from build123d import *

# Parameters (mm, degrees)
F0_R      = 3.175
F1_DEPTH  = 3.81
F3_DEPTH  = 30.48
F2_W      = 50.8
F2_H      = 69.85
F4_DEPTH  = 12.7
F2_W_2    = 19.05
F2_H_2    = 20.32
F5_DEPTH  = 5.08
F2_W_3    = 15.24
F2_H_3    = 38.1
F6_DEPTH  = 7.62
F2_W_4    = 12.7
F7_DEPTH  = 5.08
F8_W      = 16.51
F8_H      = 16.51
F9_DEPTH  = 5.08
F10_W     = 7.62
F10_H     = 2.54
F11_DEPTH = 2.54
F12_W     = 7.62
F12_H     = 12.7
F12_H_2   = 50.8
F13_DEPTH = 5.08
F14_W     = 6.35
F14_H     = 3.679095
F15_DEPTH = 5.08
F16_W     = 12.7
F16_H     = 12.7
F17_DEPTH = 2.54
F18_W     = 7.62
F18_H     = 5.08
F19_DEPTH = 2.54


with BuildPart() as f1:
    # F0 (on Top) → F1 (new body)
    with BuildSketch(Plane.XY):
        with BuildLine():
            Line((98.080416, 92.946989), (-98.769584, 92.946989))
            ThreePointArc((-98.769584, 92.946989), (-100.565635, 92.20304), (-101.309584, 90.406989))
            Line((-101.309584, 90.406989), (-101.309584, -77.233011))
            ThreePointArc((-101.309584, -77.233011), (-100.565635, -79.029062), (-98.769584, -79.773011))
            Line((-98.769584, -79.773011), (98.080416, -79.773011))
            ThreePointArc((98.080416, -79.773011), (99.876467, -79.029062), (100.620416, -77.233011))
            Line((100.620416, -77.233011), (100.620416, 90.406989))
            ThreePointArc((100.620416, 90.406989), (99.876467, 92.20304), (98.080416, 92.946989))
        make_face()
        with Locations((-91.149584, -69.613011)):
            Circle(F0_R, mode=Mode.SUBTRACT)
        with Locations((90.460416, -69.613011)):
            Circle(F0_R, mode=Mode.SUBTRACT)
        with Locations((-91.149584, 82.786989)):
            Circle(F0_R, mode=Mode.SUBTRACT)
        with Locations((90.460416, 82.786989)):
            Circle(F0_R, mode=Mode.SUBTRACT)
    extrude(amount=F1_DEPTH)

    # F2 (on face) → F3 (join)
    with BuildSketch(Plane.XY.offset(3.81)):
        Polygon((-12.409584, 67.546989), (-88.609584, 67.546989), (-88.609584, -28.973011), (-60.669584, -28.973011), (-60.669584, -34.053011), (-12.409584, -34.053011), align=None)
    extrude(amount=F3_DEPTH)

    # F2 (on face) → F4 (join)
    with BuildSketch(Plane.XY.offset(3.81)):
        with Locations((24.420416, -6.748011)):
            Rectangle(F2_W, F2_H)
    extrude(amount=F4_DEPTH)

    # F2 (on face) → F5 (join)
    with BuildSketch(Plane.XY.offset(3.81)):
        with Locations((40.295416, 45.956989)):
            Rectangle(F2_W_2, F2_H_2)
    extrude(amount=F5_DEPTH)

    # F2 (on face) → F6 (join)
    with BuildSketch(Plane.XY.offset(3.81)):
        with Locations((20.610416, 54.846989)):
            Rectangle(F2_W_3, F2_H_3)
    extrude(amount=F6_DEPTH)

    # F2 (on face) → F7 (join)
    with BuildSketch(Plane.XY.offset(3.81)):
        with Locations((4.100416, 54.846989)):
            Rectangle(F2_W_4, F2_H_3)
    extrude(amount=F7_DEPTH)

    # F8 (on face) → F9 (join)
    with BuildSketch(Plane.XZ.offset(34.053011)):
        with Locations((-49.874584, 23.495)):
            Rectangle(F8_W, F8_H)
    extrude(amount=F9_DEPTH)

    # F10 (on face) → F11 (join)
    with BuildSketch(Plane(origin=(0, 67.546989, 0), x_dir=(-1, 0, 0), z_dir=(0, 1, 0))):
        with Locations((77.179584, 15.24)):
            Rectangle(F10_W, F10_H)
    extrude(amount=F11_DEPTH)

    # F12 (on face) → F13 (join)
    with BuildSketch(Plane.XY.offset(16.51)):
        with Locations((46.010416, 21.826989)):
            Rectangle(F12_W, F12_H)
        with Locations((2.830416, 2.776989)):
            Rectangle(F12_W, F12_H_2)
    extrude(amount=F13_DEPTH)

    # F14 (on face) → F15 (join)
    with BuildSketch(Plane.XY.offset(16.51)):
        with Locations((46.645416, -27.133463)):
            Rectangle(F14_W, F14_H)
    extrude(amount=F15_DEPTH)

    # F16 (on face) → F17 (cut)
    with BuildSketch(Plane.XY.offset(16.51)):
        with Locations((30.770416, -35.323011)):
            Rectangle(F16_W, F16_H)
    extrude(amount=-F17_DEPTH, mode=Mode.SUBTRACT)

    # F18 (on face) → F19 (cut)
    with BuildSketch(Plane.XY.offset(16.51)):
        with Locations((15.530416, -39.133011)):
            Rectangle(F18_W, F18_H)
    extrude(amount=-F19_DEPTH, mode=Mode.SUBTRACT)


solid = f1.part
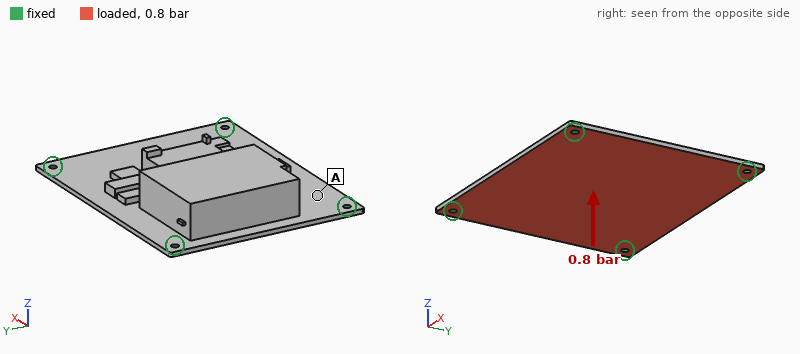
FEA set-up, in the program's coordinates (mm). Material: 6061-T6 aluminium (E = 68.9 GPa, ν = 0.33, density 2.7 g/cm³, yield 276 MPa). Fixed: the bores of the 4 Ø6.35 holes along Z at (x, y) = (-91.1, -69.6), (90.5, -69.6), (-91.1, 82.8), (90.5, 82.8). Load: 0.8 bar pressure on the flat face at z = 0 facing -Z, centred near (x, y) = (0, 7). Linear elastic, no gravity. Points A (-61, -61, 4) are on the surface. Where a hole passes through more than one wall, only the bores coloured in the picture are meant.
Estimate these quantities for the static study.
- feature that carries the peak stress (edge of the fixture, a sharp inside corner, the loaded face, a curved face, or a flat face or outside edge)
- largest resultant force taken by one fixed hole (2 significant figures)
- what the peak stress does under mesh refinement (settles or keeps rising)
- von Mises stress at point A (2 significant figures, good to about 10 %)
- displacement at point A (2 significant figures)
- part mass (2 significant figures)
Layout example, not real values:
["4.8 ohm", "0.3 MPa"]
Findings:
["edge of the fixture", "950 N", "keeps rising", "22 MPa", "0.29 mm", "1.1 kg"]
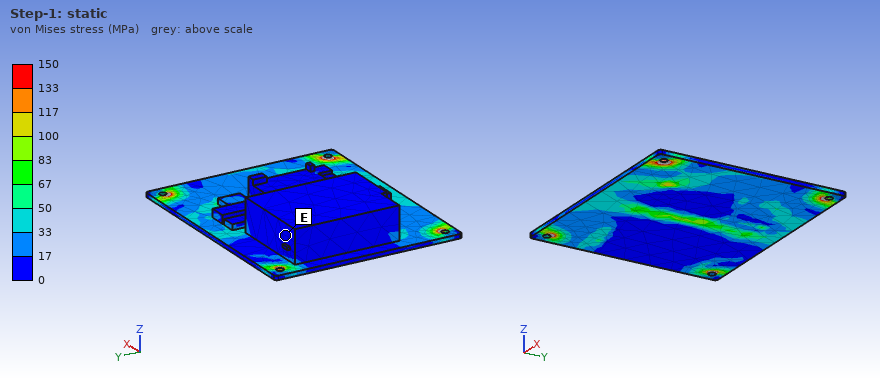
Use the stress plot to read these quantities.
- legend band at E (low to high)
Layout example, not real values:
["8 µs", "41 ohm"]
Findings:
["0 to 17 MPa"]
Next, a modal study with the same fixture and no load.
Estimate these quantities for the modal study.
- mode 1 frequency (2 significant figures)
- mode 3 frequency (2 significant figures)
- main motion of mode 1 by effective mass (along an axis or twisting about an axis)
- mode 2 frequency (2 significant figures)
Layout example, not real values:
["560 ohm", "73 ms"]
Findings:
["320 Hz", "1000 Hz", "along Z", "680 Hz"]
